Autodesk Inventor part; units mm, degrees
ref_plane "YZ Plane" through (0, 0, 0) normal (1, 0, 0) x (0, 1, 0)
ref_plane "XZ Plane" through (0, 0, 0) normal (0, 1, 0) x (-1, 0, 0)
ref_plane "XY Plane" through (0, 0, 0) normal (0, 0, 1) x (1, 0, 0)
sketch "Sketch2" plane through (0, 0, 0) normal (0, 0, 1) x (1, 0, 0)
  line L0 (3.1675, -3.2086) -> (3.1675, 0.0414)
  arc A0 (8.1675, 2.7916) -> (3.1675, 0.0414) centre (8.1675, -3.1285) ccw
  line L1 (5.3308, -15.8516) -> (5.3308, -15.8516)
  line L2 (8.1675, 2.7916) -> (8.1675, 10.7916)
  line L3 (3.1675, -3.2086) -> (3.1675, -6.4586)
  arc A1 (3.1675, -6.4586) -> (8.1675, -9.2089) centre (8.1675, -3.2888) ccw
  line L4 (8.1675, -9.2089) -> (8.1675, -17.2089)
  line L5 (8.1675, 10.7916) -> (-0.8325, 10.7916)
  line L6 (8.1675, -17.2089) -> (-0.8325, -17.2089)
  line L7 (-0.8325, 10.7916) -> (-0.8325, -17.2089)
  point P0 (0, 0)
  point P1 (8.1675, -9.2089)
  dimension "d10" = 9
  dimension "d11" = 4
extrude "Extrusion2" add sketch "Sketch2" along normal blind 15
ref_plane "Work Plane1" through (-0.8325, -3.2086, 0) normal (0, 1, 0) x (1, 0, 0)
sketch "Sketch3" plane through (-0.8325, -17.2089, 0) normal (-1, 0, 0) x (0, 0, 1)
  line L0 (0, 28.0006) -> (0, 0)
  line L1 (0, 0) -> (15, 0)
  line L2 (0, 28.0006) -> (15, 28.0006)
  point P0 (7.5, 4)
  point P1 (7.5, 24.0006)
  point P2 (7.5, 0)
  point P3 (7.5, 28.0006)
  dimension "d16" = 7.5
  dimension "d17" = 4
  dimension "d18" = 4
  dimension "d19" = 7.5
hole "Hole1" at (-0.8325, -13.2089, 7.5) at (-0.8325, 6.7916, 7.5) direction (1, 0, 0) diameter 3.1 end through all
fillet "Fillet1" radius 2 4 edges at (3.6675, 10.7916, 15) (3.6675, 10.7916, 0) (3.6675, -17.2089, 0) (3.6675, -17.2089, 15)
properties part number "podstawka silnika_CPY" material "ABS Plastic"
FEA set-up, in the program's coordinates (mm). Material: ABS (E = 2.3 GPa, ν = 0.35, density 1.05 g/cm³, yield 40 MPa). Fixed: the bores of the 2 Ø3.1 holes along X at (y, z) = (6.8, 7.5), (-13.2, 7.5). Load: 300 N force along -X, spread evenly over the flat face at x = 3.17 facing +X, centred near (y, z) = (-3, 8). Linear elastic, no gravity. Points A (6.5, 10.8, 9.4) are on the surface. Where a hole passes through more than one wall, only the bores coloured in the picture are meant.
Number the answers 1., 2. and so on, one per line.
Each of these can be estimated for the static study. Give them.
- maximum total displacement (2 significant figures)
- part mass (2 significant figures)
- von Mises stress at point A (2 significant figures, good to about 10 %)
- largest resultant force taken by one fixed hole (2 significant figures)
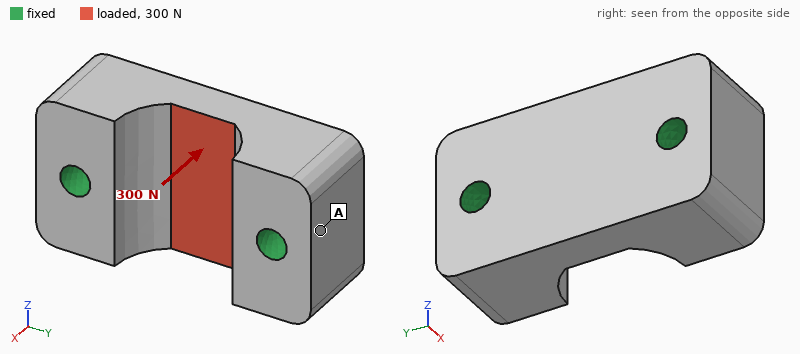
1. 45 µm
2. 3.0 g
3. 2.0 MPa
4. 160 N
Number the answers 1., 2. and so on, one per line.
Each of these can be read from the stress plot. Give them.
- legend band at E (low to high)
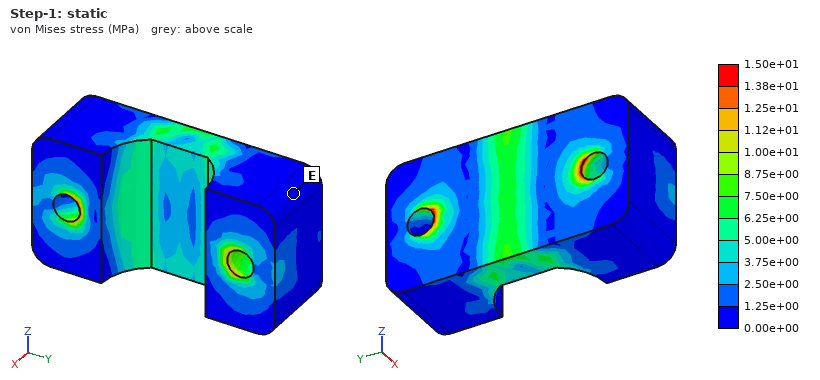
1. 0.00e+00 to 1.25e+00 MPa
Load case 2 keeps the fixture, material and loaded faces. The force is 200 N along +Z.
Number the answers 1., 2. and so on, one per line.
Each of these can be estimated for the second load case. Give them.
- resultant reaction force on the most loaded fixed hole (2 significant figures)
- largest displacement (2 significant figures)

1. 100 N
2. 29 µm
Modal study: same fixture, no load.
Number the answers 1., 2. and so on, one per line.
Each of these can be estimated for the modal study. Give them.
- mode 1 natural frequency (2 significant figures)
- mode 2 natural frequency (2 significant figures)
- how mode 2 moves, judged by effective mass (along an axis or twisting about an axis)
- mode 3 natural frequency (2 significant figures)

1. 16 kHz
2. 18 kHz
3. along X
4. 20 kHz
